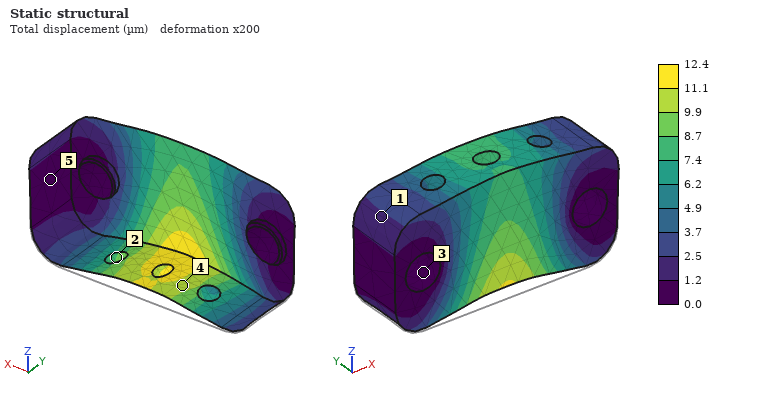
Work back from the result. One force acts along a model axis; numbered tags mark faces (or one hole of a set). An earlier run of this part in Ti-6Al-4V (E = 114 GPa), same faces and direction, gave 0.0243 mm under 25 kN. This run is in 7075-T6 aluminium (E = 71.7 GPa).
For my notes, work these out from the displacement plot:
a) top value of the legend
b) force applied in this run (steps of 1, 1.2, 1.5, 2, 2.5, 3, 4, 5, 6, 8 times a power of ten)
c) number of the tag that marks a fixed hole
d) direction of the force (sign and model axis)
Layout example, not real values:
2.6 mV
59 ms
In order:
12.4 µm
8 kN
3
+Z
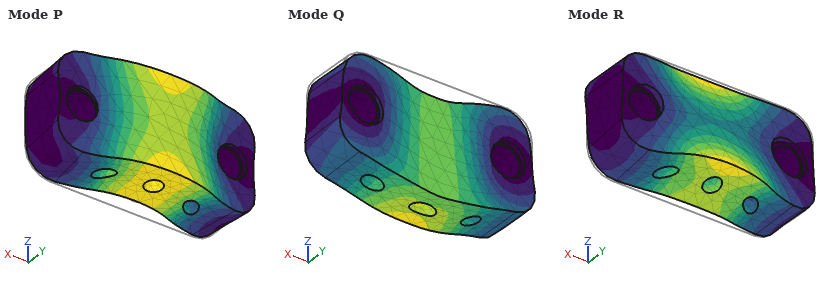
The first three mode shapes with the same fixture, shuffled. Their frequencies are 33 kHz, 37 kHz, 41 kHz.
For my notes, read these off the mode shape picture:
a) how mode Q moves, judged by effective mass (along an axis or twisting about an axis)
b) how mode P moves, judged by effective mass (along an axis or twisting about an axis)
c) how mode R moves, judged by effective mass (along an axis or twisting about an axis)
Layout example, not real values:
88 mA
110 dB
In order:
along Z
along Y
twisting about X
